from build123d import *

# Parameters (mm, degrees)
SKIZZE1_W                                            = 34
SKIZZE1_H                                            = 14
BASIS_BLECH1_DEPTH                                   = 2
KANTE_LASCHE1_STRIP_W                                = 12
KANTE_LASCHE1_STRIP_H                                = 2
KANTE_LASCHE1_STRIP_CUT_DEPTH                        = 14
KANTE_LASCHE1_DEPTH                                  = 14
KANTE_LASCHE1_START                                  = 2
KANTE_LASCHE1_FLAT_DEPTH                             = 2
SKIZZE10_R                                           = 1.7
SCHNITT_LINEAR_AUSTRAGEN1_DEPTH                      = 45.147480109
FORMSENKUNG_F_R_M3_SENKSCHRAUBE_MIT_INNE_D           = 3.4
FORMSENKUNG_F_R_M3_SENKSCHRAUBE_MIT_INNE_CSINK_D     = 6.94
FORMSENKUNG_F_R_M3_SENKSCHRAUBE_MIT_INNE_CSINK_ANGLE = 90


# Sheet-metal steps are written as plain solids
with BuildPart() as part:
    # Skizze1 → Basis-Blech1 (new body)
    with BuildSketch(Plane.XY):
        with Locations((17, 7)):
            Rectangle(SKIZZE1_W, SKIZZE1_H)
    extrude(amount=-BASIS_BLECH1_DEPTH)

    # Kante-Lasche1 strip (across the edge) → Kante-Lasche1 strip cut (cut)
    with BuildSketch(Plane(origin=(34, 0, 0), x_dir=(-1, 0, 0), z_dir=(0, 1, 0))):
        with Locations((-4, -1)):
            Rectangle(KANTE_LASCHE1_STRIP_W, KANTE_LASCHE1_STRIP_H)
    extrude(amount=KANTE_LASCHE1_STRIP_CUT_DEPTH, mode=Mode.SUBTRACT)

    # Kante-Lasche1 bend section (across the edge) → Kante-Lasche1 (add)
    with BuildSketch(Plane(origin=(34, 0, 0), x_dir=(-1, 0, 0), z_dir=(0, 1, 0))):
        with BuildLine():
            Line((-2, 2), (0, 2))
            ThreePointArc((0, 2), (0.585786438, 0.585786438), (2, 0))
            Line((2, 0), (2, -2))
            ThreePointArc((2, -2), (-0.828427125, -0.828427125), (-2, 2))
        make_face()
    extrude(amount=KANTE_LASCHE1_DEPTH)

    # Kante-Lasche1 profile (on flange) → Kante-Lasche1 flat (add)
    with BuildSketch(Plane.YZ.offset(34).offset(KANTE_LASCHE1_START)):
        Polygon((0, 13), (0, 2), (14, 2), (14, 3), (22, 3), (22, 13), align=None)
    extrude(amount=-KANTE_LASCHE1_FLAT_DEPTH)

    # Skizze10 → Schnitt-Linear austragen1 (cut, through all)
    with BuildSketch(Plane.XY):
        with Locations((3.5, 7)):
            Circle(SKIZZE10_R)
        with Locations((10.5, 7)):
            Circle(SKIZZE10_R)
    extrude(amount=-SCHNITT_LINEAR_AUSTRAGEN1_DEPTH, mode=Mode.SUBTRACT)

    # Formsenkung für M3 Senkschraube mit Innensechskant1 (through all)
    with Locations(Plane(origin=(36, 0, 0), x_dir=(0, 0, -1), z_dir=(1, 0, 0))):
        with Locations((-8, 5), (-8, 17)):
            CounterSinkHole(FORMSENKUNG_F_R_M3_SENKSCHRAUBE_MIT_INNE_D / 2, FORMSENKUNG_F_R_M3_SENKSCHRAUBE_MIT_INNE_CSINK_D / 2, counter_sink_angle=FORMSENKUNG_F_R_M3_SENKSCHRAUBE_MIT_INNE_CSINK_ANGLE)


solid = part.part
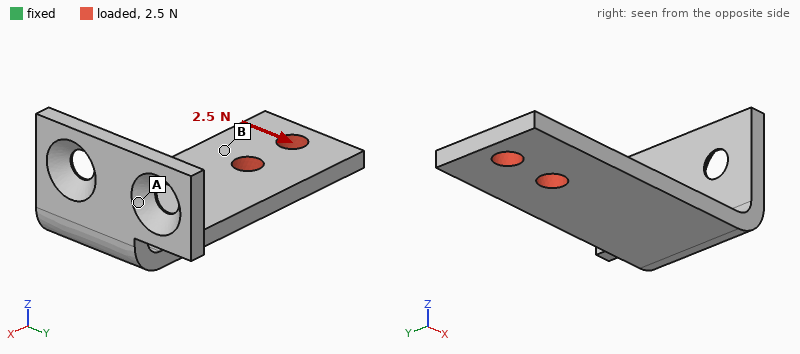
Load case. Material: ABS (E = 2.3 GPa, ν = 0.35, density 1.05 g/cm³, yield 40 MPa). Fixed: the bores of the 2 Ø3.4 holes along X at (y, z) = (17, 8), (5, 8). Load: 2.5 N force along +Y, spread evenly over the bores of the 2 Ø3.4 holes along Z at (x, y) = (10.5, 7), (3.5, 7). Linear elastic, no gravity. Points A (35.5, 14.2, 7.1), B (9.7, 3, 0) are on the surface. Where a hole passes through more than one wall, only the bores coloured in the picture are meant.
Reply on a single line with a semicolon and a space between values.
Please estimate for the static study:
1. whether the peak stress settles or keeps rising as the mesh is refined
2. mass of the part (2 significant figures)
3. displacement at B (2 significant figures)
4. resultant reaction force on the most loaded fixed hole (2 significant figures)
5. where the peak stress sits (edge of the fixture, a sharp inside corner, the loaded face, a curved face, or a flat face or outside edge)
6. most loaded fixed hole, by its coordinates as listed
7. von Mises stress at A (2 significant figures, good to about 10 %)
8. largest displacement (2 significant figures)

keeps rising; 1.4 g; 0.38 mm; 9.5 N; edge of the fixture; (5, 8); 3.9 MPa; 0.54 mm
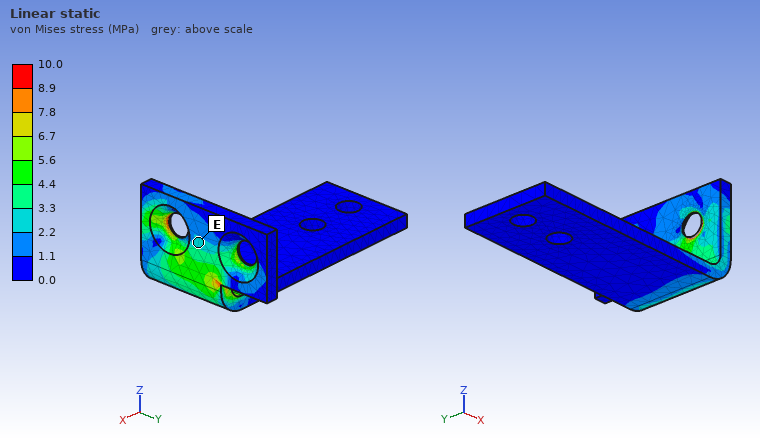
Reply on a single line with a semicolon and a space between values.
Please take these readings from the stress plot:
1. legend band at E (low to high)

2.2 to 3.3 MPa
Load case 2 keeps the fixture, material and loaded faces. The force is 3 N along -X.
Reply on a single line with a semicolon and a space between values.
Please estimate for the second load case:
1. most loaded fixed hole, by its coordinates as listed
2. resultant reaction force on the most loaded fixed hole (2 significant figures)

(5, 8); 2.7 N
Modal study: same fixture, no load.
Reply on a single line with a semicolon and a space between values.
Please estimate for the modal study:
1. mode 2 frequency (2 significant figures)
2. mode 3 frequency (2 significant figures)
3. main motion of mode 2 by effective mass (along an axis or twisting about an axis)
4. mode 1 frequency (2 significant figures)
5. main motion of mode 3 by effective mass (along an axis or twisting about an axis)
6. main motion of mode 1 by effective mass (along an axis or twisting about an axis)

550 Hz; 1300 Hz; along Y; 260 Hz; along X; along Z
